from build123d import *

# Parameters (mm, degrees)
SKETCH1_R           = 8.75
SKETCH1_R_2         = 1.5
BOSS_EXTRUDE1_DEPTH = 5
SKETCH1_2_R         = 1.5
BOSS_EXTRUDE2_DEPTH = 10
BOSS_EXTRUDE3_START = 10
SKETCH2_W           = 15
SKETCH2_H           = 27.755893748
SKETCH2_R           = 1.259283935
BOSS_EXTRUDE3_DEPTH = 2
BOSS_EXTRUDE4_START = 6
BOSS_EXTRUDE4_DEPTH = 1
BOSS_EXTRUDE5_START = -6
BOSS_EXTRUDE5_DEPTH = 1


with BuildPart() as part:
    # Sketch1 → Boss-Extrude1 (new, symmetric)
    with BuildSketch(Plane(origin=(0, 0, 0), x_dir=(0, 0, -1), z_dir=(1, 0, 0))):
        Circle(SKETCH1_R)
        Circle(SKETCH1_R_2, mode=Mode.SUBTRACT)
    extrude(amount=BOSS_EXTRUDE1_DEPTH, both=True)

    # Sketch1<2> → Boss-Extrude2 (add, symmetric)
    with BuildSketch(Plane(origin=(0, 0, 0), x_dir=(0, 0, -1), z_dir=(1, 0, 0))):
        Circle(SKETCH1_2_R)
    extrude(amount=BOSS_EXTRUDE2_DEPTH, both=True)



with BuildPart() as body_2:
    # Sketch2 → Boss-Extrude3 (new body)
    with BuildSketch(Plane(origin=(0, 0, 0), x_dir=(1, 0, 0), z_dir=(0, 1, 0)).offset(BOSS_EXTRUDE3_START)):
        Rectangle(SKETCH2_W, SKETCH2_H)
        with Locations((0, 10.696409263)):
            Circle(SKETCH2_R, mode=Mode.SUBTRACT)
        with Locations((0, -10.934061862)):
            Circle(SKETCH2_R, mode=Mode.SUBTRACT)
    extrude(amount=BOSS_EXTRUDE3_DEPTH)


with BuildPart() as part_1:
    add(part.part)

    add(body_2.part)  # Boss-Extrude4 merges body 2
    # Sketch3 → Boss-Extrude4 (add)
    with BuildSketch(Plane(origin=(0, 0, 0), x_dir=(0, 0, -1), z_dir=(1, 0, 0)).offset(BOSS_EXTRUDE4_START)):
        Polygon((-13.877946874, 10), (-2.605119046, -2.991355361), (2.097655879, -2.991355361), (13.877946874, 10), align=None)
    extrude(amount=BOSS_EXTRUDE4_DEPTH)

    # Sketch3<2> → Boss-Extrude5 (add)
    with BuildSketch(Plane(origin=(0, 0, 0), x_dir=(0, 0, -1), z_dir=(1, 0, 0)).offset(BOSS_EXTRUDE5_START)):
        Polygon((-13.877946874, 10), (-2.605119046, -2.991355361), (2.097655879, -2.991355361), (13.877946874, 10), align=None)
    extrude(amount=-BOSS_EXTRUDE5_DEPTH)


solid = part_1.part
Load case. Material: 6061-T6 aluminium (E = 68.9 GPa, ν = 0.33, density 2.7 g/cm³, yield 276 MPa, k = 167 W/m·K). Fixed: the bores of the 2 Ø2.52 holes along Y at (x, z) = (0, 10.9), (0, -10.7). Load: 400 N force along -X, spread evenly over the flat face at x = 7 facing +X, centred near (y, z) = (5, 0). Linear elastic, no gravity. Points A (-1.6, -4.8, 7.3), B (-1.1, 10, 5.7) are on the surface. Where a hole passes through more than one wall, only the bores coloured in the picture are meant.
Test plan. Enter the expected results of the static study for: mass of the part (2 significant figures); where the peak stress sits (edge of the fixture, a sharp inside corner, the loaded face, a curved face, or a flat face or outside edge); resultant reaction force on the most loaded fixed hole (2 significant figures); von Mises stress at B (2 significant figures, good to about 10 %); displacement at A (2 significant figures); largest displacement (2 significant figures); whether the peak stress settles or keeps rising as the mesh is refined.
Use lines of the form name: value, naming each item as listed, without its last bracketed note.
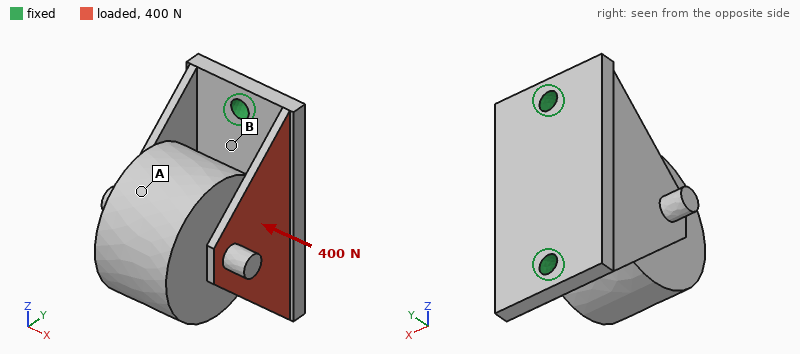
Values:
mass of the part: 10.0 g
where the peak stress sits: edge of the fixture
resultant reaction force on the most loaded fixed hole: 200 N
von Mises stress at B: 26 MPa
displacement at A: 0.16 mm
largest displacement: 0.18 mm
whether the peak stress settles or keeps rising as the mesh is refined: keeps rising
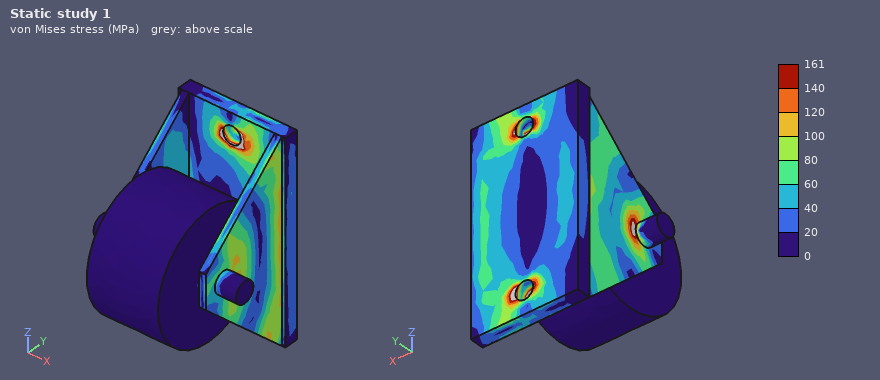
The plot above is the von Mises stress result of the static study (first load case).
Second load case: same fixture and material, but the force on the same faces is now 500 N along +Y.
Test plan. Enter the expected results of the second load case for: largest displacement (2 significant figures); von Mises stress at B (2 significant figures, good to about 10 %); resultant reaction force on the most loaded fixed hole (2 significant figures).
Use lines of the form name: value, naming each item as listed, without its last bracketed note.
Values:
largest displacement: 0.13 mm
von Mises stress at B: 46 MPa
resultant reaction force on the most loaded fixed hole: 250 N
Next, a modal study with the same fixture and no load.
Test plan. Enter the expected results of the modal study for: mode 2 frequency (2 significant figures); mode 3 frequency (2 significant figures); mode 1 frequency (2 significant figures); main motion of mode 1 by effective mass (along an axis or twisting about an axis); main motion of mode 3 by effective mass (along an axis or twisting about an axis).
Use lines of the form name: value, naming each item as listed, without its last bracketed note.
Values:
mode 2 frequency: 4300 Hz
mode 3 frequency: 7600 Hz
mode 1 frequency: 2100 Hz
main motion of mode 1 by effective mass: along X
main motion of mode 3 by effective mass: along Z
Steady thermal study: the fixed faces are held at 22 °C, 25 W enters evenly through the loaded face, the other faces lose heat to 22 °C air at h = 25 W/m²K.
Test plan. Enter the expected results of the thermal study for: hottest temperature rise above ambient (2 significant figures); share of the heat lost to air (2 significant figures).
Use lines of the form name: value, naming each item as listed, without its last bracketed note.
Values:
hottest temperature rise above ambient: 46 K
share of the heat lost to air: 6.1 %
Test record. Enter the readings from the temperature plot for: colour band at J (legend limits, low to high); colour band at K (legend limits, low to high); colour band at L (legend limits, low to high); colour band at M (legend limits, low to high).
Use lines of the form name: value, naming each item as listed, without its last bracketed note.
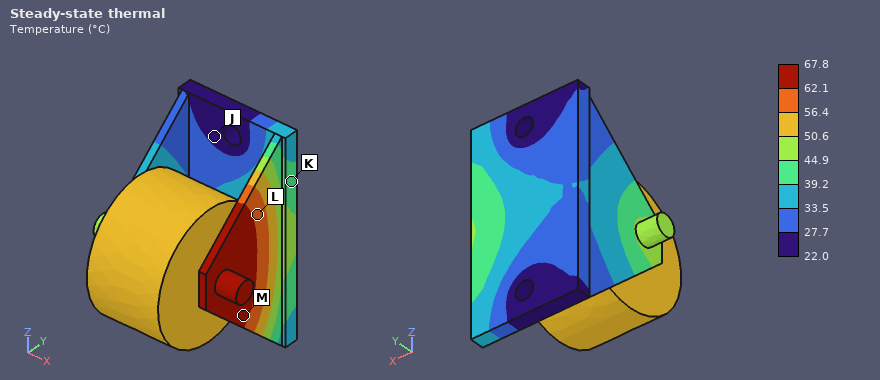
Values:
colour band at J: 22.0 to 27.7 °C
colour band at K: 39.2 to 44.9 °C
colour band at L: 56.4 to 62.1 °C
colour band at M: 62.1 to 67.8 °C
